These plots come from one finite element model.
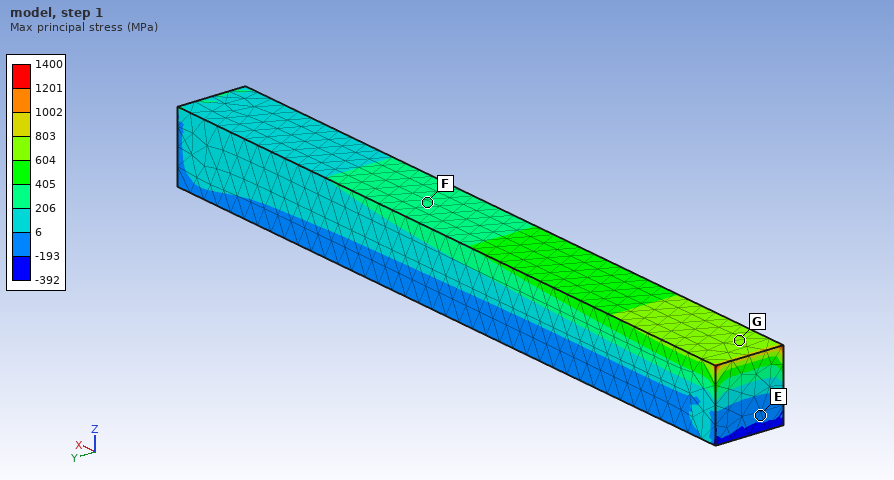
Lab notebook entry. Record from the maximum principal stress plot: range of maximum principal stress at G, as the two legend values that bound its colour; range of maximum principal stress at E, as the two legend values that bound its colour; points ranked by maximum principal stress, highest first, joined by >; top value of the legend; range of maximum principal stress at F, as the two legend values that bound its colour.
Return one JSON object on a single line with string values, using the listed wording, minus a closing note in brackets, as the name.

{"range of maximum principal stress at G, as the two legend values that bound its colour": "604 to 803 MPa", "range of maximum principal stress at E, as the two legend values that bound its colour": "-193 to 6 MPa", "points ranked by maximum principal stress, highest first, joined by >": "G > F > E", "top value of the legend": "1400 MPa", "range of maximum principal stress at F, as the two legend values that bound its colour": "206 to 405 MPa"}
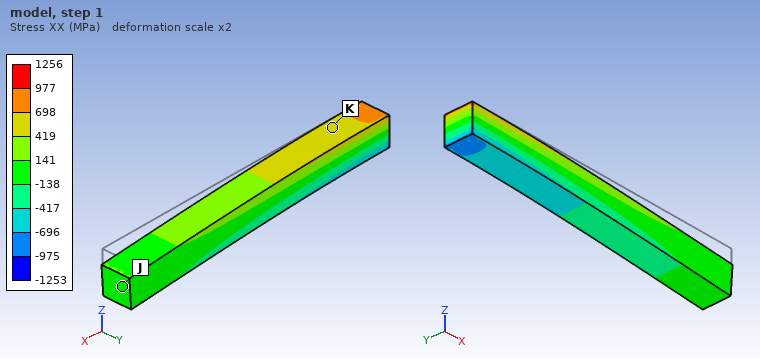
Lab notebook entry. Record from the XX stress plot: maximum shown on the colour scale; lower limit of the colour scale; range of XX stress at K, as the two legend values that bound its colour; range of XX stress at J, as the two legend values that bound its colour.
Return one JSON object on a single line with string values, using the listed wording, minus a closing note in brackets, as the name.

{"maximum shown on the colour scale": "1256 MPa", "lower limit of the colour scale": "-1253 MPa", "range of XX stress at K, as the two legend values that bound its colour": "419 to 698 MPa", "range of XX stress at J, as the two legend values that bound its colour": "-138 to 141 MPa"}
